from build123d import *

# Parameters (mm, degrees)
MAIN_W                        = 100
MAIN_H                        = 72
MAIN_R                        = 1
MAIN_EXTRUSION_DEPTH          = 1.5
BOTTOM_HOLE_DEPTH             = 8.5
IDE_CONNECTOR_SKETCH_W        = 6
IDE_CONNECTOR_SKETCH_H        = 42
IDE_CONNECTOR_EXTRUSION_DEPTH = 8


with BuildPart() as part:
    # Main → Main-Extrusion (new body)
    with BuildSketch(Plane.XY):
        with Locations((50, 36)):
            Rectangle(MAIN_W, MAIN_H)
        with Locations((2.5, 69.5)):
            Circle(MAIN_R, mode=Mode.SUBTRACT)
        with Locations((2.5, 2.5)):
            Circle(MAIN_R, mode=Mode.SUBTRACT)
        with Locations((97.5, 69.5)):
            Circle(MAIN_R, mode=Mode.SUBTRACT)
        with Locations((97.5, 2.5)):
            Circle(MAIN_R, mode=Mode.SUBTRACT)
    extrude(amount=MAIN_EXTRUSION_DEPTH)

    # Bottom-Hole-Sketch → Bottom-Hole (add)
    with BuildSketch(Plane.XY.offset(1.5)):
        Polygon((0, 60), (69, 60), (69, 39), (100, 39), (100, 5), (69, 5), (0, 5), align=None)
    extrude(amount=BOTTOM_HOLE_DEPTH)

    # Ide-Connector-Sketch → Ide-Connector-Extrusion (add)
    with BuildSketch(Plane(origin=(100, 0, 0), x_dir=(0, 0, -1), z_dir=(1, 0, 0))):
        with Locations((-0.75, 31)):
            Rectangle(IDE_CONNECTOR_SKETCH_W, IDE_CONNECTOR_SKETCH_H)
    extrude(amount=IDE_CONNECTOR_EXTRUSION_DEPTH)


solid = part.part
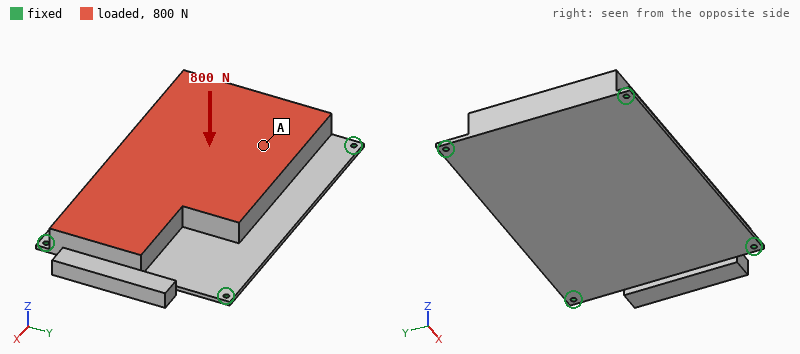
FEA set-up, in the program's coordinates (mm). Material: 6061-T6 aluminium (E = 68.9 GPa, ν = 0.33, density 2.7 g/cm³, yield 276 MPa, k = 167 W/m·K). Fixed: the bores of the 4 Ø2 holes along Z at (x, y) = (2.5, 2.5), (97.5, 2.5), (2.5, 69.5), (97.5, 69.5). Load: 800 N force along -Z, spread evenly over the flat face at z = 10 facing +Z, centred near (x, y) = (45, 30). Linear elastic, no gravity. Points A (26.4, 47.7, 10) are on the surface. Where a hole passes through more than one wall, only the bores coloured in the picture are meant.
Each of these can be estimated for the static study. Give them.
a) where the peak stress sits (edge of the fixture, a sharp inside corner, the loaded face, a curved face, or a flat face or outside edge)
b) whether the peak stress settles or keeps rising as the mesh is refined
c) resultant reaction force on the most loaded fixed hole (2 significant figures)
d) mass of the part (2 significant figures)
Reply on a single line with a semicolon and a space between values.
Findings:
edge of the fixture; keeps rising; 470 N; 150 g
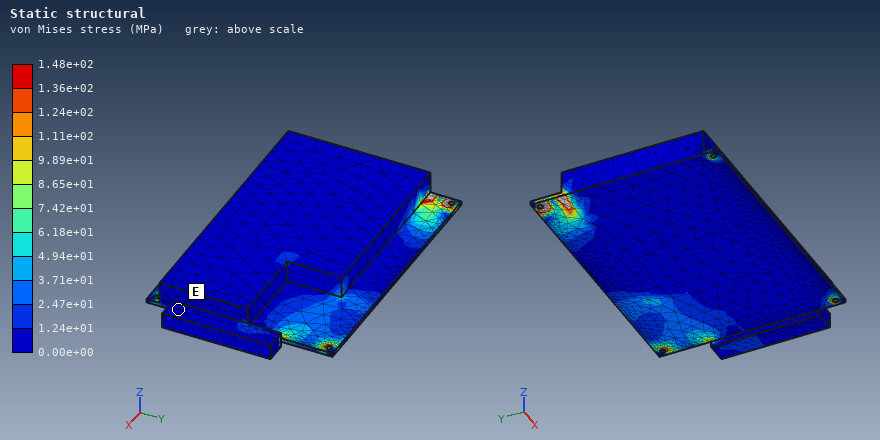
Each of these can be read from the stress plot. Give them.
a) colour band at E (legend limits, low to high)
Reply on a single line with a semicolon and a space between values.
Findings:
0.00e+00 to 1.24e+01 MPa
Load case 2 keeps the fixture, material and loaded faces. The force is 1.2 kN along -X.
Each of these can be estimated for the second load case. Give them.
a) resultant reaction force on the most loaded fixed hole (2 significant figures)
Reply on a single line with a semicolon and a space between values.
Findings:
470 N
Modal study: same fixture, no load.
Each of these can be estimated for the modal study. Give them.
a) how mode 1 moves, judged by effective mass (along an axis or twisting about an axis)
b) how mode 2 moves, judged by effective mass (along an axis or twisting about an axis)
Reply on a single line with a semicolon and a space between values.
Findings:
along Z; twisting about Y
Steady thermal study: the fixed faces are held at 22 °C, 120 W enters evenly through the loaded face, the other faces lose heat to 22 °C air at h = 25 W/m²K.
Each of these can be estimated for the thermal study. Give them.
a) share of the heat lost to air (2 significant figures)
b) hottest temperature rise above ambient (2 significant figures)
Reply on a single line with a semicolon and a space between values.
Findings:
21 %; 86 K
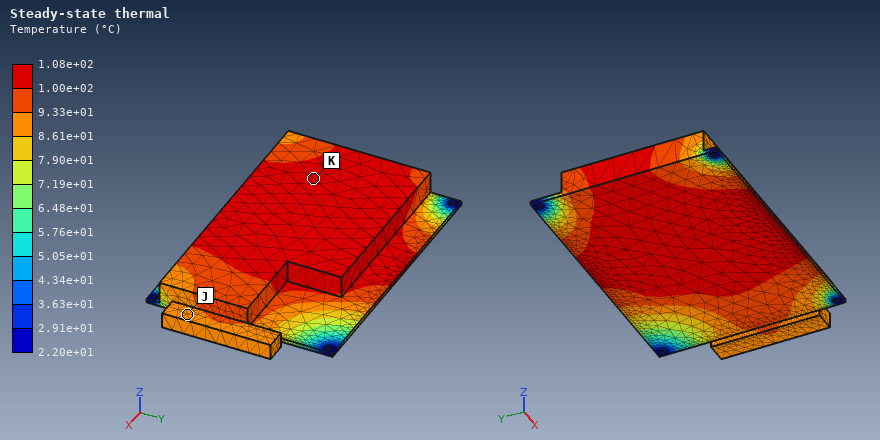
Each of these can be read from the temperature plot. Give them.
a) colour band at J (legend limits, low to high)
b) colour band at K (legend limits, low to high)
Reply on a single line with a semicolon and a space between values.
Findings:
8.61e+01 to 9.33e+01 °C; 1.00e+02 to 1.08e+02 °C
